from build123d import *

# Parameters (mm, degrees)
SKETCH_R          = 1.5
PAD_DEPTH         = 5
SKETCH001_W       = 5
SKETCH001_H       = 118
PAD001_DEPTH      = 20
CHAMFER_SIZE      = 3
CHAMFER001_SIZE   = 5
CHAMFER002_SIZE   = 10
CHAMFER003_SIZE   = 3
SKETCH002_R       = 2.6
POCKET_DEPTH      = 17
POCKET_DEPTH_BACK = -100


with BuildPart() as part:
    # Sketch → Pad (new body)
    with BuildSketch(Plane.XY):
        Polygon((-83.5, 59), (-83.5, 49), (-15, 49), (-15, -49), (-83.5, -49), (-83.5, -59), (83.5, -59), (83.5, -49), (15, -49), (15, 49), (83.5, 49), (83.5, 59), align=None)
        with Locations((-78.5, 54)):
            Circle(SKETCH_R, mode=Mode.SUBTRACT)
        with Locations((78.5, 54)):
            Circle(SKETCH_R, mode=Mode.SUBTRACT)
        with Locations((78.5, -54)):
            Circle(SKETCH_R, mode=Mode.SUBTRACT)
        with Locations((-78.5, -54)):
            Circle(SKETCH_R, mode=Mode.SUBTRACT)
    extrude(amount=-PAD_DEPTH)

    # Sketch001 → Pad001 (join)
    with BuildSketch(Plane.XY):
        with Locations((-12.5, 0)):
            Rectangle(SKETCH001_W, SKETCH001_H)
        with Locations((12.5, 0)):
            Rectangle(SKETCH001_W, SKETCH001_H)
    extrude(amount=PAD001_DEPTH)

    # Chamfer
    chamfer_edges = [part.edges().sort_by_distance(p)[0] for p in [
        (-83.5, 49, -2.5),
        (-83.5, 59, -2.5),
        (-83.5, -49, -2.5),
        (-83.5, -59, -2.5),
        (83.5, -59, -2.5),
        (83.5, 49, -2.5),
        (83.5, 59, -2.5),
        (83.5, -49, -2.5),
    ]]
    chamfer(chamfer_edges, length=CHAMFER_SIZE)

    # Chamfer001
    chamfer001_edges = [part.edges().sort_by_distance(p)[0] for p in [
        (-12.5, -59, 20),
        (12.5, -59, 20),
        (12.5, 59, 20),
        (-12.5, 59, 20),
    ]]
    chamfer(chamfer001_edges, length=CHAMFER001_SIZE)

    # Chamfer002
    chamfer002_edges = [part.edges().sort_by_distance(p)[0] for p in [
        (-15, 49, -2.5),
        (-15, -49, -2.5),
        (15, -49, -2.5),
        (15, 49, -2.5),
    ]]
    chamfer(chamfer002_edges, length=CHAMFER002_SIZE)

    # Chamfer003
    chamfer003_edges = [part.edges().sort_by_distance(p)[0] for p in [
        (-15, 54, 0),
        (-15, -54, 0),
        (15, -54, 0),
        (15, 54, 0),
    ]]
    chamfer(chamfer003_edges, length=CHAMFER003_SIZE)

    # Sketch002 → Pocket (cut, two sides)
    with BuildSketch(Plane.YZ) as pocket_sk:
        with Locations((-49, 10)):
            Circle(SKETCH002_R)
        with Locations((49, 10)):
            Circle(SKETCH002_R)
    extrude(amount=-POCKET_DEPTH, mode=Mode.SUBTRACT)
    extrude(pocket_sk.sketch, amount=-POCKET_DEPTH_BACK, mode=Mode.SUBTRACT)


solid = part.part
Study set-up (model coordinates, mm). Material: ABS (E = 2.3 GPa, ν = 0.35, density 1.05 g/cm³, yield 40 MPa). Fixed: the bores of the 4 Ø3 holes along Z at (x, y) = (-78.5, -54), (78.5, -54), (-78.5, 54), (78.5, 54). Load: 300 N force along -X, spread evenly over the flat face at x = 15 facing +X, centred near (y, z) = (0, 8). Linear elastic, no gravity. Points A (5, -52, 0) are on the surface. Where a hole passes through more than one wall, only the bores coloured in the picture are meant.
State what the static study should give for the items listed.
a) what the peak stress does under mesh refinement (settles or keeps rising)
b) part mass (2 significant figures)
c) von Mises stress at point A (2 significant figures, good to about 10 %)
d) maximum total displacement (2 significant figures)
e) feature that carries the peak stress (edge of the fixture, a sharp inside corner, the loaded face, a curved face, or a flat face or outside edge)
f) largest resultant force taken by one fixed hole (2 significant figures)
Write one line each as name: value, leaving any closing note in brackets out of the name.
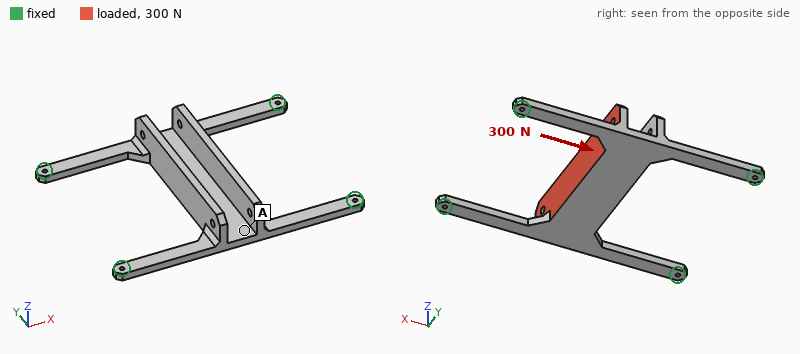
what the peak stress does under mesh refinement: keeps rising
part mass: 58 g
von Mises stress at point A: 3.1 MPa
maximum total displacement: 1.2 mm
feature that carries the peak stress: edge of the fixture
largest resultant force taken by one fixed hole: 78 N
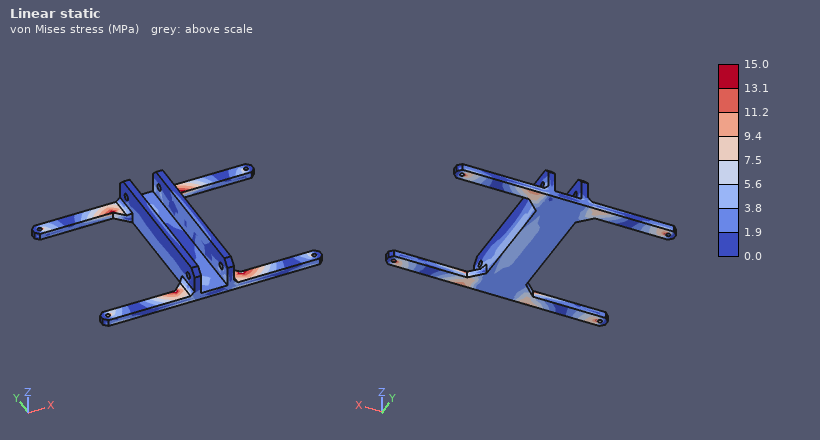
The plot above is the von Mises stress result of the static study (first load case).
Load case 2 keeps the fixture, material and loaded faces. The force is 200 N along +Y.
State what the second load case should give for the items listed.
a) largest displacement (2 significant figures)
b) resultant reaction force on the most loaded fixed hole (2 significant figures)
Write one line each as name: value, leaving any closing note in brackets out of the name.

largest displacement: 1.9 mm
resultant reaction force on the most loaded fixed hole: 73 N
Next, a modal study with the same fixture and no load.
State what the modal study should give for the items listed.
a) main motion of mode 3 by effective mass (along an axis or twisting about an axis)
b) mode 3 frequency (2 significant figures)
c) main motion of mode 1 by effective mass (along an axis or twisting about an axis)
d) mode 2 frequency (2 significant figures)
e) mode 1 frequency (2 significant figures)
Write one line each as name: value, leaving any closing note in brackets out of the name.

main motion of mode 3 by effective mass: along Y
mode 3 frequency: 290 Hz
main motion of mode 1 by effective mass: along Z
mode 2 frequency: 220 Hz
mode 1 frequency: 150 Hz
